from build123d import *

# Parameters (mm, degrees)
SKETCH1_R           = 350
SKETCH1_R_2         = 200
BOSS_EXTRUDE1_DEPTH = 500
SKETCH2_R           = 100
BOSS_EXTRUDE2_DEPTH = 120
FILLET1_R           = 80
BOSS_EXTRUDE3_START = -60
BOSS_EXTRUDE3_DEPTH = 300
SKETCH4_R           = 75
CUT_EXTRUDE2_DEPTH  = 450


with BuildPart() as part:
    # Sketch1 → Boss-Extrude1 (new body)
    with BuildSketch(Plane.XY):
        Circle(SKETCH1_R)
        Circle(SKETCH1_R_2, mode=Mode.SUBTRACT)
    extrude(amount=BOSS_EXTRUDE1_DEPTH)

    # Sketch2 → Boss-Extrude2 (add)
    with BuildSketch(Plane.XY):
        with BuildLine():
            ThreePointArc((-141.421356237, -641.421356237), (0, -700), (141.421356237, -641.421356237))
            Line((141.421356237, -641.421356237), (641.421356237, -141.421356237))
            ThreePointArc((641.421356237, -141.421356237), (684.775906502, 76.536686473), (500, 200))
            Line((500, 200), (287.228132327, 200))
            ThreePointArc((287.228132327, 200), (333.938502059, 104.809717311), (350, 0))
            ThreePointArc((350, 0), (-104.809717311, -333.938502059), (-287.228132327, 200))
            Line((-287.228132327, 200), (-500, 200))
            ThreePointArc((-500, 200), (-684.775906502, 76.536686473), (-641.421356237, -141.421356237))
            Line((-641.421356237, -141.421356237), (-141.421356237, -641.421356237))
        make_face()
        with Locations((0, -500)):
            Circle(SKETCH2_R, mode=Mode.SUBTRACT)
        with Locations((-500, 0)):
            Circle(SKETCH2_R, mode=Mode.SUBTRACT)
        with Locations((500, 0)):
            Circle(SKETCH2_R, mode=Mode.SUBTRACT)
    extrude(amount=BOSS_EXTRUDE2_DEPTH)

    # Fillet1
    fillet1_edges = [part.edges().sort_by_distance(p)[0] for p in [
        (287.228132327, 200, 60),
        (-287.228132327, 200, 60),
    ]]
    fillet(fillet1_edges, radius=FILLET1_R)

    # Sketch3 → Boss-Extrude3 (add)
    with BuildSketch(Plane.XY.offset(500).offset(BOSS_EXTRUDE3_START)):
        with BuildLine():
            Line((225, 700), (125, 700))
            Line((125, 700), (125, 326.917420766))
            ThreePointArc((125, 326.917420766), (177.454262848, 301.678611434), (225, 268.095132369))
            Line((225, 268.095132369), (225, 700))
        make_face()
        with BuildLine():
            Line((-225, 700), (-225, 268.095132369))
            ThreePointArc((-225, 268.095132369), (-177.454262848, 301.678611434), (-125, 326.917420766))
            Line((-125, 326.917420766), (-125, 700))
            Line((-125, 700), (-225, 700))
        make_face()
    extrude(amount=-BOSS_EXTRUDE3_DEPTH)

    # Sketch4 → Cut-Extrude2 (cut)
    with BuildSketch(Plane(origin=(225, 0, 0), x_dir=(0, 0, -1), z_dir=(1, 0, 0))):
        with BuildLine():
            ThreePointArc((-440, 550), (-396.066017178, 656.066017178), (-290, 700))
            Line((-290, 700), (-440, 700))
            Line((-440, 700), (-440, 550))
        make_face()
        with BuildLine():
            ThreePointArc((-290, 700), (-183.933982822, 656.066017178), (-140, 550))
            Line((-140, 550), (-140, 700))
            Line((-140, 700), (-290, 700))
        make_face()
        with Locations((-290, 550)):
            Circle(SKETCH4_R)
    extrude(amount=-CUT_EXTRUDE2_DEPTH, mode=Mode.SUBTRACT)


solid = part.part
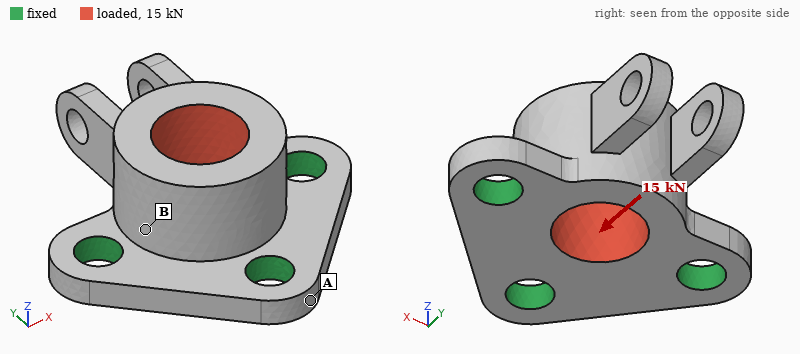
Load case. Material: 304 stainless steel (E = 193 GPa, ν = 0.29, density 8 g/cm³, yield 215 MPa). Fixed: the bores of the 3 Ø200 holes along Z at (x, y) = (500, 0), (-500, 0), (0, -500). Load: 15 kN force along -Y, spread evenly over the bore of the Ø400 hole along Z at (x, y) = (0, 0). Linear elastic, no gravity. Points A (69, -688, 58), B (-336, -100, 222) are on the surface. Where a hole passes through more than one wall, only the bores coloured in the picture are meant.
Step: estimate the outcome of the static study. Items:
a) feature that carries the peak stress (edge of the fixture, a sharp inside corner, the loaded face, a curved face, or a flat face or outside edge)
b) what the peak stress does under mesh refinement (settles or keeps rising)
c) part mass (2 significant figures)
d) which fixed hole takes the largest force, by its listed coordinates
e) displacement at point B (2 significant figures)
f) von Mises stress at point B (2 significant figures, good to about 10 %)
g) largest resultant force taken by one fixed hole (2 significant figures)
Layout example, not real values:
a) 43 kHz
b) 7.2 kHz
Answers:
a) edge of the fixture
b) keeps rising
c) 1600 kg
d) (0, -500)
e) 0.59 µm
f) 0.14 MPa
g) 8.9 kN
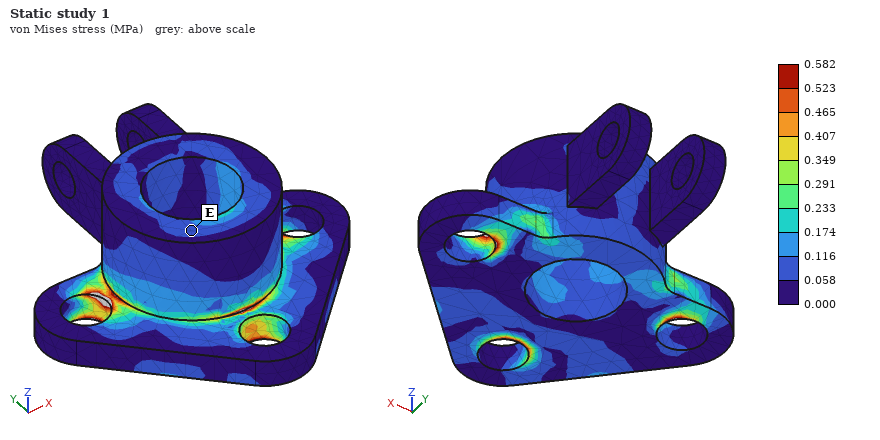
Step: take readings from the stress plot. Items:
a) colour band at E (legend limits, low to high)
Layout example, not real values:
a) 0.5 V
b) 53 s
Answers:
a) 0.058 to 0.116 MPa
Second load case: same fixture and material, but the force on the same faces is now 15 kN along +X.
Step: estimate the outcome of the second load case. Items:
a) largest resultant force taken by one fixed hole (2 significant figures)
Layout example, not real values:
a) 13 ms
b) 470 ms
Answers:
a) 7.2 kN
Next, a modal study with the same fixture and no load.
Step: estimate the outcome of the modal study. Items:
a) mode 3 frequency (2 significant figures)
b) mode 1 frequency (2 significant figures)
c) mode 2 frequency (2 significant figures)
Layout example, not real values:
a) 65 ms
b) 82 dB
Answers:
a) 520 Hz
b) 350 Hz
c) 500 Hz
